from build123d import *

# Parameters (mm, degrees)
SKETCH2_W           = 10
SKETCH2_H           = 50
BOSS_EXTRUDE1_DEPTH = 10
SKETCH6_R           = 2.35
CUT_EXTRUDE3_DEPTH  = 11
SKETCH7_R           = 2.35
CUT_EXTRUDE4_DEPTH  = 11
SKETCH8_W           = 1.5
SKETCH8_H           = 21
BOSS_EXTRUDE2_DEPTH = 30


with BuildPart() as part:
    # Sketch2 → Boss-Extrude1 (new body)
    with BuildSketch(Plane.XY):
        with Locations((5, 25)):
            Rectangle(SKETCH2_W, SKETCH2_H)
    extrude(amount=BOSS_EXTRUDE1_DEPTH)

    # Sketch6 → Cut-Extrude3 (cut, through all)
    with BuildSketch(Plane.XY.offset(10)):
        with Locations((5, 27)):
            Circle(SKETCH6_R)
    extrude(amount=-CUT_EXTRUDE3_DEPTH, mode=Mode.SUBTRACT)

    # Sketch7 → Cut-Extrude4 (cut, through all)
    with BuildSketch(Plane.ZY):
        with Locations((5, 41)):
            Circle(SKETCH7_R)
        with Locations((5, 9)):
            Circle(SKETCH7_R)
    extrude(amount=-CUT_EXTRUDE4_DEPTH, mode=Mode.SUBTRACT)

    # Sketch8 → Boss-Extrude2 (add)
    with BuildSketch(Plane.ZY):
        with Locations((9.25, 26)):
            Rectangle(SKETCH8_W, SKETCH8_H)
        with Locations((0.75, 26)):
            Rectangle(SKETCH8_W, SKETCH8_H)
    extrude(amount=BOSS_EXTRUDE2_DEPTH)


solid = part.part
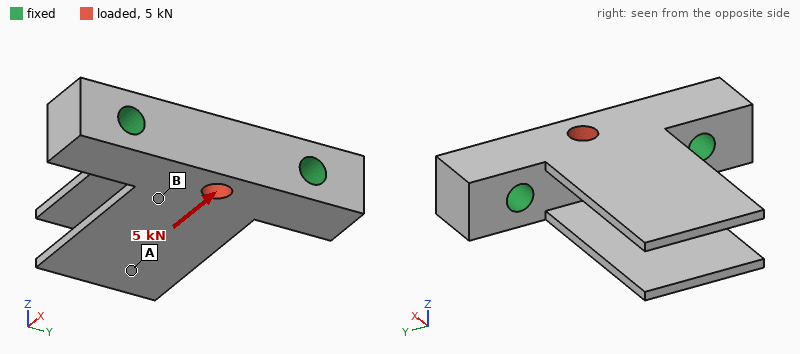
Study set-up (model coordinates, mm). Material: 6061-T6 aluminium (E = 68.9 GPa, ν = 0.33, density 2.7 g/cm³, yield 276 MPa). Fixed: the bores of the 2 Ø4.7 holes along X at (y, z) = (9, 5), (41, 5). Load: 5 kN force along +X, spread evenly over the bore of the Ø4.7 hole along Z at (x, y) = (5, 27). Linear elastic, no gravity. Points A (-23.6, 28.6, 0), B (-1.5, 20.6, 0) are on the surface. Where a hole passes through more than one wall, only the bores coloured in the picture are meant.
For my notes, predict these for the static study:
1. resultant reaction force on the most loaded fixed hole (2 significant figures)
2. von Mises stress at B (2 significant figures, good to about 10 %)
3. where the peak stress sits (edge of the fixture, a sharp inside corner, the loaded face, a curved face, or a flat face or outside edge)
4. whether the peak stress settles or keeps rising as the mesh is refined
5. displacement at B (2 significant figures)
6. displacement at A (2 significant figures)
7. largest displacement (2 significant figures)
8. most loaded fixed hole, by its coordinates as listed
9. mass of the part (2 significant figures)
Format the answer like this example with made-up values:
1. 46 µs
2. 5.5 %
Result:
1. 2.9 kN
2. 46 MPa
3. edge of the fixture
4. keeps rising
5. 15 µm
6. 14 µm
7. 23 µm
8. (41, 5)
9. 17 g
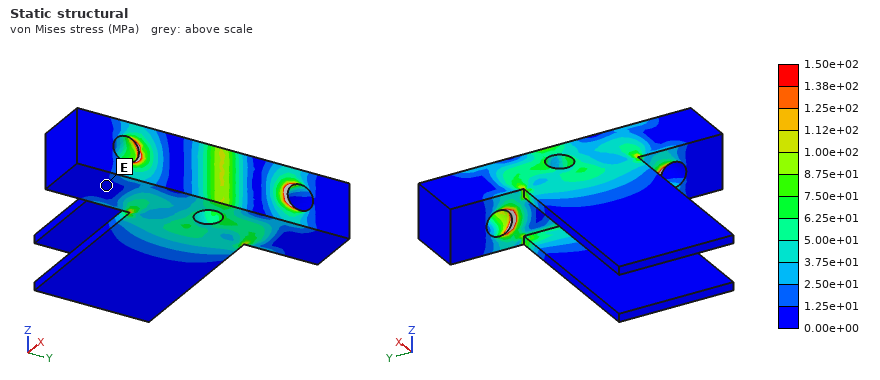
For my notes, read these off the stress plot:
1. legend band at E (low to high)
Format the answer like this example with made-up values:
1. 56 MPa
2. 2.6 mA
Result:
1. 0.00e+00 to 1.25e+01 MPa
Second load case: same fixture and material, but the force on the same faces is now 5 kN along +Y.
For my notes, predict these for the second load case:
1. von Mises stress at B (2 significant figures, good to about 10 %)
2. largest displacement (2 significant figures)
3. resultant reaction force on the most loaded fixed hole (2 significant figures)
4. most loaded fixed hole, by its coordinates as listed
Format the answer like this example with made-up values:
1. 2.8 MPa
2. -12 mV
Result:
1. 5.0 MPa
2. 5.8 µm
3. 2.8 kN
4. (41, 5)
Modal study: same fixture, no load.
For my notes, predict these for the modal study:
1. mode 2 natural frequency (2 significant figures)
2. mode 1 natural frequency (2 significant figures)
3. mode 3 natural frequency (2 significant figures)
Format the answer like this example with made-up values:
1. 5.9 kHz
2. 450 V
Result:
1. 1300 Hz
2. 1300 Hz
3. 4200 Hz
